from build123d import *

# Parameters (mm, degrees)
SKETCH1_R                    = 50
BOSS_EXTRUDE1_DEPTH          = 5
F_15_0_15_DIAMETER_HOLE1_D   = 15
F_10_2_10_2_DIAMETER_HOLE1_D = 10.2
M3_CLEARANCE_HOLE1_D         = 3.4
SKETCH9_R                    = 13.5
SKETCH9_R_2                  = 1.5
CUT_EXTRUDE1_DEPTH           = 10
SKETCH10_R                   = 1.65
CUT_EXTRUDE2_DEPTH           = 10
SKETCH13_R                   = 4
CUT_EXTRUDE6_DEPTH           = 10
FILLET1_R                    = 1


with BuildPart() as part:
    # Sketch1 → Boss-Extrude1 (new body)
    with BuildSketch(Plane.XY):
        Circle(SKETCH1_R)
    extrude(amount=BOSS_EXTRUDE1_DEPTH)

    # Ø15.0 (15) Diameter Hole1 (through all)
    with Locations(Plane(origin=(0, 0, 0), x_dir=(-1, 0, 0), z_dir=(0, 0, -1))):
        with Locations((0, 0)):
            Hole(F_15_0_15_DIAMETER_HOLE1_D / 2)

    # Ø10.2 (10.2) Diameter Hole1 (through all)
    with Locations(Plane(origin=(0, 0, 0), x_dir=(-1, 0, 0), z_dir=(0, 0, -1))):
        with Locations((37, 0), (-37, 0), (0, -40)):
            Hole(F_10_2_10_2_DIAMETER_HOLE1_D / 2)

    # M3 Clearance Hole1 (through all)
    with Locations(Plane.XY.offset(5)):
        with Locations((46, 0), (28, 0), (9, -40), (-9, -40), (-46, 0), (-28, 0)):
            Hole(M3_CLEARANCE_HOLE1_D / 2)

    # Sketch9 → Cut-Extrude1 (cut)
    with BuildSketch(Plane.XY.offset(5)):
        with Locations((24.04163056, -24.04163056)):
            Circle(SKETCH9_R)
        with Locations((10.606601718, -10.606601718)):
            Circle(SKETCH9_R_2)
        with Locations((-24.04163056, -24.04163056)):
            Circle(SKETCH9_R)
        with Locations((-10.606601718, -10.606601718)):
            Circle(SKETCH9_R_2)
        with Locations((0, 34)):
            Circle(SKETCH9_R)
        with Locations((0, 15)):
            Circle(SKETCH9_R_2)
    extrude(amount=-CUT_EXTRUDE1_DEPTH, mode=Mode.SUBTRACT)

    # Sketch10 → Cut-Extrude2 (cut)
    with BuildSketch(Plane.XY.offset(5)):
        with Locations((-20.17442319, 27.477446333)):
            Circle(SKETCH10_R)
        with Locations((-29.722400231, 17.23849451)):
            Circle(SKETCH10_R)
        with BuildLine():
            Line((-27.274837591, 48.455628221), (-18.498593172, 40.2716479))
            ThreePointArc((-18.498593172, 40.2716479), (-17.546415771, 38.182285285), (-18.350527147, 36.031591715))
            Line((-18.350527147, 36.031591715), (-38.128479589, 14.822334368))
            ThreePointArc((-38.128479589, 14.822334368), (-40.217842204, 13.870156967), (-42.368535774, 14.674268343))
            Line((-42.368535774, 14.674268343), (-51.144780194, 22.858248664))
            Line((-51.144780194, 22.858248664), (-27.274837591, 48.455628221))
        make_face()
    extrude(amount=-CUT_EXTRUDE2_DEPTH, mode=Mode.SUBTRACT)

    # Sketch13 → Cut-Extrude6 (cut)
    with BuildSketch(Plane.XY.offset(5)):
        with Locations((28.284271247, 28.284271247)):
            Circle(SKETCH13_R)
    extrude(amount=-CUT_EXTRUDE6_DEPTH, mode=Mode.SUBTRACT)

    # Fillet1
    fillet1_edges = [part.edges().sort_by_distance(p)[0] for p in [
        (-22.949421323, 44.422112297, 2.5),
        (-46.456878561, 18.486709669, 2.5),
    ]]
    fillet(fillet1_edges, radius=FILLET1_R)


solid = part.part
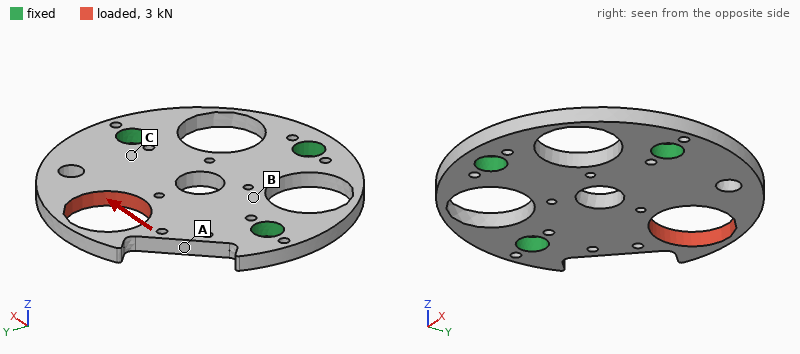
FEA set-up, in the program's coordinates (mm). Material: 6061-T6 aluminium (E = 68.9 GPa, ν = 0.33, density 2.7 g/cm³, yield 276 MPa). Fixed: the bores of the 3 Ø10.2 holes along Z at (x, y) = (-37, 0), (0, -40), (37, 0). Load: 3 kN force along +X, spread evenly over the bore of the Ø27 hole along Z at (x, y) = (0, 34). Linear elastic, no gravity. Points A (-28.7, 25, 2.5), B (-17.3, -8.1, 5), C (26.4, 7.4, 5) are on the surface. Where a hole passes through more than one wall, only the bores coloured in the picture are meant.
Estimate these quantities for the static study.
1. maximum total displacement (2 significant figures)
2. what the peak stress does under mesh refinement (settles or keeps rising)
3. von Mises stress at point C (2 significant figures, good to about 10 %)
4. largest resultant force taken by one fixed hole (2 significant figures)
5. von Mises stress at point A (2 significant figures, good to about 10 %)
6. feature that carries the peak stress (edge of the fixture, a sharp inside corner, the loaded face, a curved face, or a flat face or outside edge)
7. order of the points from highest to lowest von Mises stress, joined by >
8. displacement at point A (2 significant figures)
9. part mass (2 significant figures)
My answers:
54 µm
keeps rising
14 MPa
2.0 kN
33 MPa
a sharp inside corner
A > C > B
10 µm
70 g
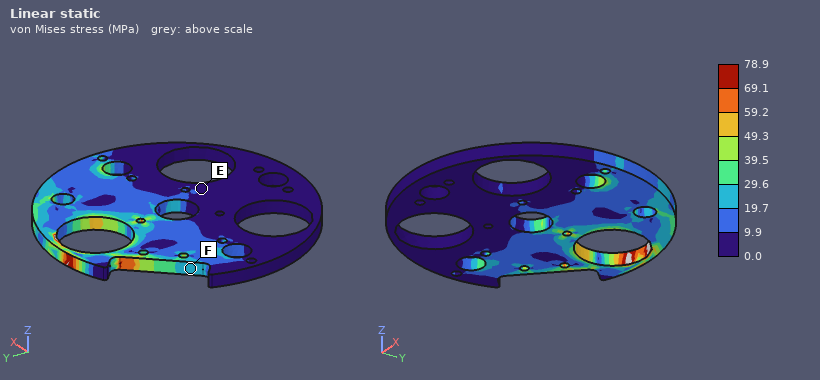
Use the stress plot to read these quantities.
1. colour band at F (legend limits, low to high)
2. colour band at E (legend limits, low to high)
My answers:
19.7 to 29.6 MPa
0.0 to 9.9 MPa
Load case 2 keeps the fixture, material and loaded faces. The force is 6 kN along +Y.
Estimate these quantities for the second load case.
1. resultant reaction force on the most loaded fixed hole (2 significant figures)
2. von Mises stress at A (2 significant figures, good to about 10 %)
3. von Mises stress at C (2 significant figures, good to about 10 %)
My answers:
2.7 kN
37 MPa
27 MPa
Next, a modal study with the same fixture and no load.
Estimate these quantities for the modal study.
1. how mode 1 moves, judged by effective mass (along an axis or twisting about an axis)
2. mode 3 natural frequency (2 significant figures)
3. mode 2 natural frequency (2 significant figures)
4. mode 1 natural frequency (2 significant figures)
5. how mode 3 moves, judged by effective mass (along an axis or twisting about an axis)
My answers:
along Z
6000 Hz
4600 Hz
2300 Hz
along Z
